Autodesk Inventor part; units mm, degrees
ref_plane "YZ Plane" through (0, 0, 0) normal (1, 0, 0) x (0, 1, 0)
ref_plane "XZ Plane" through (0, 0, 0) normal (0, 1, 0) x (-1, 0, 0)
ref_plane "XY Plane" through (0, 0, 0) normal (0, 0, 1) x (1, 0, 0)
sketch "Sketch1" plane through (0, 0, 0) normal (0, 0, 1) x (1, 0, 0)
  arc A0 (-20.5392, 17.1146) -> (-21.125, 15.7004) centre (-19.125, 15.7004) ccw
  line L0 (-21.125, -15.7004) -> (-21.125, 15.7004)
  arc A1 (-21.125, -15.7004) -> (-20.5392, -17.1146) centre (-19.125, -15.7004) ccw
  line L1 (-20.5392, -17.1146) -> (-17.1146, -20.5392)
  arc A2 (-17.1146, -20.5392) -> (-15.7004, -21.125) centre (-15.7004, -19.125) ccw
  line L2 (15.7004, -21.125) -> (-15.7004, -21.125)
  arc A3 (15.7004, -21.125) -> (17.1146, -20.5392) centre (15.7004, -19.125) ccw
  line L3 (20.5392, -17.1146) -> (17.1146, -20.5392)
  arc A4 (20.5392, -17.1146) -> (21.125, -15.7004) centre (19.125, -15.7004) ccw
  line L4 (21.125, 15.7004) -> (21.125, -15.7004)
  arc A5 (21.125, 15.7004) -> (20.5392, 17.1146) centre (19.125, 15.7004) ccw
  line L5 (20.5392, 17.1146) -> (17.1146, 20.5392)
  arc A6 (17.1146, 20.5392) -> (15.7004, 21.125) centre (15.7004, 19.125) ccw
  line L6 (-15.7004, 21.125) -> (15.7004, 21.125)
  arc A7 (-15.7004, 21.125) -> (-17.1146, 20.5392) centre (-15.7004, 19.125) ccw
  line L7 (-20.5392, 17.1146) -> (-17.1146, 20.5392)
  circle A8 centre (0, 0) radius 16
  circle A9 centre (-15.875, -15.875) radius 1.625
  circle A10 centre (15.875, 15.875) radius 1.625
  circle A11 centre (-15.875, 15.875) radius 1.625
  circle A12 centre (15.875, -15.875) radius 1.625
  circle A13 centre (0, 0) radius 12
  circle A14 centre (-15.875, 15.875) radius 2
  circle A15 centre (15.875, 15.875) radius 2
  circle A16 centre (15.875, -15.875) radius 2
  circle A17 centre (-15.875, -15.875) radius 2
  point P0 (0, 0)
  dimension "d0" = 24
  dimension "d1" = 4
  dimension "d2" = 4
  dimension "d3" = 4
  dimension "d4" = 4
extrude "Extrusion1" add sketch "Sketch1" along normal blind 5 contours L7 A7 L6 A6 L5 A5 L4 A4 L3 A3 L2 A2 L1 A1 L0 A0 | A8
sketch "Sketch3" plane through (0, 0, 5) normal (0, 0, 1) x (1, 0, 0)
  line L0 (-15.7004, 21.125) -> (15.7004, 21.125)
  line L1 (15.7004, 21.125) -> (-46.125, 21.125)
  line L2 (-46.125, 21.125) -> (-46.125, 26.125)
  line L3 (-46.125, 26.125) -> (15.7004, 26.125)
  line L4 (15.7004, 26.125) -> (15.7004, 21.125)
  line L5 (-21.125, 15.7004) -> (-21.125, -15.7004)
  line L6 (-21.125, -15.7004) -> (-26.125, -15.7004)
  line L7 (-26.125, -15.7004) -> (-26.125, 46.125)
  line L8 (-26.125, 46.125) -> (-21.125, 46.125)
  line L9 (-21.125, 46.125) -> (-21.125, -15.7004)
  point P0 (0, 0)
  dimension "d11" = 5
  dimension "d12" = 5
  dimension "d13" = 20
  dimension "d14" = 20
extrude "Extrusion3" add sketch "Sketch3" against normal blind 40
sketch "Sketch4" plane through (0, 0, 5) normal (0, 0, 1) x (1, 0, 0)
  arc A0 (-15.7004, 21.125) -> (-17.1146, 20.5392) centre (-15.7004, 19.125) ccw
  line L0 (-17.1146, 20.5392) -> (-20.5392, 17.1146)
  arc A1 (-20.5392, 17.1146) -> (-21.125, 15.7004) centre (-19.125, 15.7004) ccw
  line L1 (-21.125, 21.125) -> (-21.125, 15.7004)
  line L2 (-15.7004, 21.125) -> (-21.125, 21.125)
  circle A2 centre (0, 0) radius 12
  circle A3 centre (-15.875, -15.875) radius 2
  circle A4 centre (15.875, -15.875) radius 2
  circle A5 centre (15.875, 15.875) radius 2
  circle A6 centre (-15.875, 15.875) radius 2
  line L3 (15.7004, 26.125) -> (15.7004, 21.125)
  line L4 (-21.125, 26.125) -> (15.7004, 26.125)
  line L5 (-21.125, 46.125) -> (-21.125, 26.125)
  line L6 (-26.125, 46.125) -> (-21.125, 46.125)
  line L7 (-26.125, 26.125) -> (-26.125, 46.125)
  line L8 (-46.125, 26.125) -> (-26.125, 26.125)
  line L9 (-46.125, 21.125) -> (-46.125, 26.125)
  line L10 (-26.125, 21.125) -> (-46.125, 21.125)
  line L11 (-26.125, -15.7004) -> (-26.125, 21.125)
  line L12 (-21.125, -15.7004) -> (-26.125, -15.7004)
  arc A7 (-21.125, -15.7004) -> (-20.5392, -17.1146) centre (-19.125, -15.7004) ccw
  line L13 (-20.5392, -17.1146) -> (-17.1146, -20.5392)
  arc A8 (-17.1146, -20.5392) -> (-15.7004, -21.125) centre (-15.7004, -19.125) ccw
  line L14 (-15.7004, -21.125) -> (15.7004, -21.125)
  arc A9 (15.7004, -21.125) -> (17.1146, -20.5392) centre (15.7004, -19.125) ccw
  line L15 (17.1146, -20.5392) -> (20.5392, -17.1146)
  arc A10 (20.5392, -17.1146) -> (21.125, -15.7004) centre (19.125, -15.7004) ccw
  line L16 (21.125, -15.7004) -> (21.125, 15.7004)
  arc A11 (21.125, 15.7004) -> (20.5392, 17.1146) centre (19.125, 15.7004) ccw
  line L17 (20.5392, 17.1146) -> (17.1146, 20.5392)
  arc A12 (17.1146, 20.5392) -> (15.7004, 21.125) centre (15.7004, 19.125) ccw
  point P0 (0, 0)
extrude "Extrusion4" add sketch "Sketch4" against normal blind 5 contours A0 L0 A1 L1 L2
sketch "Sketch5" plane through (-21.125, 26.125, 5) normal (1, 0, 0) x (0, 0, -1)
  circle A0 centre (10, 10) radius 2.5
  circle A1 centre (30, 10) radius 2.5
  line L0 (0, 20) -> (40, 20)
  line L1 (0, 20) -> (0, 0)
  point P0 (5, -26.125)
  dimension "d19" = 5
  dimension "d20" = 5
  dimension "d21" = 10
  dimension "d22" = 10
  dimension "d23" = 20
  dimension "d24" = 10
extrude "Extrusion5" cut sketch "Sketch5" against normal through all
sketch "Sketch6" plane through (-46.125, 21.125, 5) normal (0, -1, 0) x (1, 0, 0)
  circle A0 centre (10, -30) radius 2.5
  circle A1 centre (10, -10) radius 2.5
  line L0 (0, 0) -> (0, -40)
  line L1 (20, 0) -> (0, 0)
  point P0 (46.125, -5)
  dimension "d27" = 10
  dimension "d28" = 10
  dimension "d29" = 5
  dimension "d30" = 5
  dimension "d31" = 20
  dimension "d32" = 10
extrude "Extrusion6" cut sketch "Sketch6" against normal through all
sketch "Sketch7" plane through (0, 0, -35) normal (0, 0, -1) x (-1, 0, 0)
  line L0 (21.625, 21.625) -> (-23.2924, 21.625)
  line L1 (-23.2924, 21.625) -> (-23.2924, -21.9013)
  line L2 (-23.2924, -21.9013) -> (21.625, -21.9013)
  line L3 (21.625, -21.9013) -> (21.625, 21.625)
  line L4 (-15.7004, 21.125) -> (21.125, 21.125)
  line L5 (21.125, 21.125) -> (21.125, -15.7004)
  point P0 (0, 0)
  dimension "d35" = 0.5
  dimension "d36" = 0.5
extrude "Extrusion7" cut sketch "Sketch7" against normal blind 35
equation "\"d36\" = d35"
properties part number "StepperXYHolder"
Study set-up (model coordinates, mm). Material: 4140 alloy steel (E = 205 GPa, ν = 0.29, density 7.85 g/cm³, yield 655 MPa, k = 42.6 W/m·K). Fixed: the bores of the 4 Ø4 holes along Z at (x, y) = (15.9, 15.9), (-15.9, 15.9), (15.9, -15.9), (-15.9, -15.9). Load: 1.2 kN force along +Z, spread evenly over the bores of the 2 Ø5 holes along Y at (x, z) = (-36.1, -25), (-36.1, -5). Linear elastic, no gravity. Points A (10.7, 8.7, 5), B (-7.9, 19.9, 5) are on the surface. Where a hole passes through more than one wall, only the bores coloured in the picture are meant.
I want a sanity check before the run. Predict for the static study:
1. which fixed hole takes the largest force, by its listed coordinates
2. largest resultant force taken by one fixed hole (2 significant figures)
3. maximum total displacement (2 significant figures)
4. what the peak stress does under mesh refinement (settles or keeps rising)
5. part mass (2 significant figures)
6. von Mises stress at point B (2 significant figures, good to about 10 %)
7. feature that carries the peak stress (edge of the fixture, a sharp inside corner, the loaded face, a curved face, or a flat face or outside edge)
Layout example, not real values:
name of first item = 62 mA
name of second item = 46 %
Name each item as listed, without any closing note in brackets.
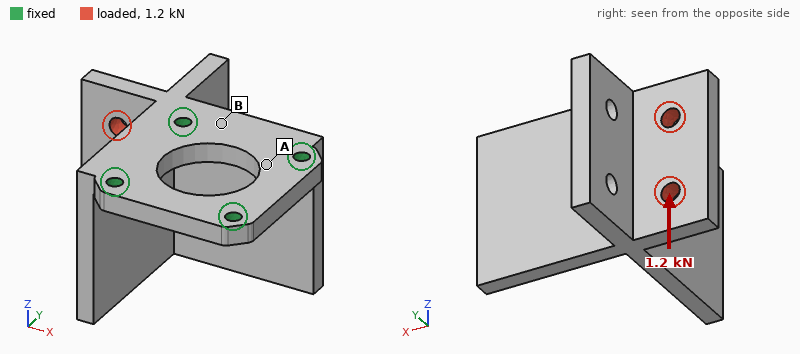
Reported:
which fixed hole takes the largest force, by its listed coordinates = (-15.9, 15.9)
largest resultant force taken by one fixed hole = 2.1 kN
maximum total displacement = 26 µm
what the peak stress does under mesh refinement = keeps rising
part mass = 220 g
von Mises stress at point B = 18 MPa
feature that carries the peak stress = edge of the fixture
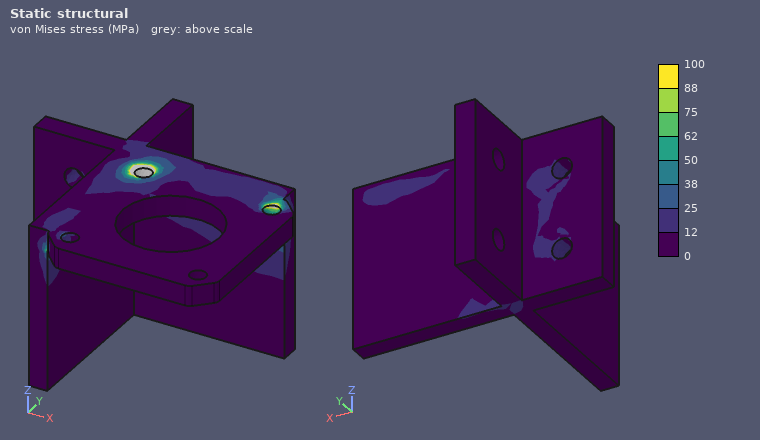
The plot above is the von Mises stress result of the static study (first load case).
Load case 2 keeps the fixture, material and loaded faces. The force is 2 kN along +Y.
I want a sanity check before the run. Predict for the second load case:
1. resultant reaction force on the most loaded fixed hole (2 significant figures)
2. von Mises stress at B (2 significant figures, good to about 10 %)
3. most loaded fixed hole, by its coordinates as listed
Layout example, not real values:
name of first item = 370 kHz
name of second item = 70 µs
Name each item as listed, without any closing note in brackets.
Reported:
resultant reaction force on the most loaded fixed hole = 1.8 kN
von Mises stress at B = 27 MPa
most loaded fixed hole, by its coordinates as listed = (-15.9, -15.9)
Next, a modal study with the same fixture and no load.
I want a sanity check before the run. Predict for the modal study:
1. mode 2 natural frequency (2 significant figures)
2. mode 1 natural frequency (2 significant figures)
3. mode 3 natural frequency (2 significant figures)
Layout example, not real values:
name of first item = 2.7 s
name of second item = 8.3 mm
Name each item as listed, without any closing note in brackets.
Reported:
mode 2 natural frequency = 3700 Hz
mode 1 natural frequency = 3300 Hz
mode 3 natural frequency = 5000 Hz
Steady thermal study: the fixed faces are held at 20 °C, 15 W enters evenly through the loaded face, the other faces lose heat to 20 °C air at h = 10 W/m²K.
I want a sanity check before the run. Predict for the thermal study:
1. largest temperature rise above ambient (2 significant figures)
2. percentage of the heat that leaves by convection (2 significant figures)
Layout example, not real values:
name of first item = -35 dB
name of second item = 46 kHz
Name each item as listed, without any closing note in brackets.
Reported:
largest temperature rise above ambient = 52 K
percentage of the heat that leaves by convection = 16 %
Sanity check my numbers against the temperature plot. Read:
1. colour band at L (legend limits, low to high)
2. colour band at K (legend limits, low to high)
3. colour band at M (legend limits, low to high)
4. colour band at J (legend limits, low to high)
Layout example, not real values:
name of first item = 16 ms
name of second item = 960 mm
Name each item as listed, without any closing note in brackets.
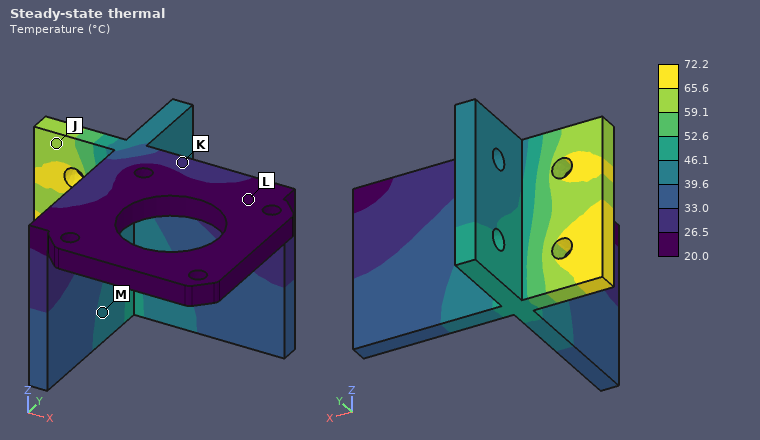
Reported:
colour band at L = 20.0 to 26.5 °C
colour band at K = 26.5 to 33.0 °C
colour band at M = 39.6 to 46.1 °C
colour band at J = 59.1 to 65.6 °C
